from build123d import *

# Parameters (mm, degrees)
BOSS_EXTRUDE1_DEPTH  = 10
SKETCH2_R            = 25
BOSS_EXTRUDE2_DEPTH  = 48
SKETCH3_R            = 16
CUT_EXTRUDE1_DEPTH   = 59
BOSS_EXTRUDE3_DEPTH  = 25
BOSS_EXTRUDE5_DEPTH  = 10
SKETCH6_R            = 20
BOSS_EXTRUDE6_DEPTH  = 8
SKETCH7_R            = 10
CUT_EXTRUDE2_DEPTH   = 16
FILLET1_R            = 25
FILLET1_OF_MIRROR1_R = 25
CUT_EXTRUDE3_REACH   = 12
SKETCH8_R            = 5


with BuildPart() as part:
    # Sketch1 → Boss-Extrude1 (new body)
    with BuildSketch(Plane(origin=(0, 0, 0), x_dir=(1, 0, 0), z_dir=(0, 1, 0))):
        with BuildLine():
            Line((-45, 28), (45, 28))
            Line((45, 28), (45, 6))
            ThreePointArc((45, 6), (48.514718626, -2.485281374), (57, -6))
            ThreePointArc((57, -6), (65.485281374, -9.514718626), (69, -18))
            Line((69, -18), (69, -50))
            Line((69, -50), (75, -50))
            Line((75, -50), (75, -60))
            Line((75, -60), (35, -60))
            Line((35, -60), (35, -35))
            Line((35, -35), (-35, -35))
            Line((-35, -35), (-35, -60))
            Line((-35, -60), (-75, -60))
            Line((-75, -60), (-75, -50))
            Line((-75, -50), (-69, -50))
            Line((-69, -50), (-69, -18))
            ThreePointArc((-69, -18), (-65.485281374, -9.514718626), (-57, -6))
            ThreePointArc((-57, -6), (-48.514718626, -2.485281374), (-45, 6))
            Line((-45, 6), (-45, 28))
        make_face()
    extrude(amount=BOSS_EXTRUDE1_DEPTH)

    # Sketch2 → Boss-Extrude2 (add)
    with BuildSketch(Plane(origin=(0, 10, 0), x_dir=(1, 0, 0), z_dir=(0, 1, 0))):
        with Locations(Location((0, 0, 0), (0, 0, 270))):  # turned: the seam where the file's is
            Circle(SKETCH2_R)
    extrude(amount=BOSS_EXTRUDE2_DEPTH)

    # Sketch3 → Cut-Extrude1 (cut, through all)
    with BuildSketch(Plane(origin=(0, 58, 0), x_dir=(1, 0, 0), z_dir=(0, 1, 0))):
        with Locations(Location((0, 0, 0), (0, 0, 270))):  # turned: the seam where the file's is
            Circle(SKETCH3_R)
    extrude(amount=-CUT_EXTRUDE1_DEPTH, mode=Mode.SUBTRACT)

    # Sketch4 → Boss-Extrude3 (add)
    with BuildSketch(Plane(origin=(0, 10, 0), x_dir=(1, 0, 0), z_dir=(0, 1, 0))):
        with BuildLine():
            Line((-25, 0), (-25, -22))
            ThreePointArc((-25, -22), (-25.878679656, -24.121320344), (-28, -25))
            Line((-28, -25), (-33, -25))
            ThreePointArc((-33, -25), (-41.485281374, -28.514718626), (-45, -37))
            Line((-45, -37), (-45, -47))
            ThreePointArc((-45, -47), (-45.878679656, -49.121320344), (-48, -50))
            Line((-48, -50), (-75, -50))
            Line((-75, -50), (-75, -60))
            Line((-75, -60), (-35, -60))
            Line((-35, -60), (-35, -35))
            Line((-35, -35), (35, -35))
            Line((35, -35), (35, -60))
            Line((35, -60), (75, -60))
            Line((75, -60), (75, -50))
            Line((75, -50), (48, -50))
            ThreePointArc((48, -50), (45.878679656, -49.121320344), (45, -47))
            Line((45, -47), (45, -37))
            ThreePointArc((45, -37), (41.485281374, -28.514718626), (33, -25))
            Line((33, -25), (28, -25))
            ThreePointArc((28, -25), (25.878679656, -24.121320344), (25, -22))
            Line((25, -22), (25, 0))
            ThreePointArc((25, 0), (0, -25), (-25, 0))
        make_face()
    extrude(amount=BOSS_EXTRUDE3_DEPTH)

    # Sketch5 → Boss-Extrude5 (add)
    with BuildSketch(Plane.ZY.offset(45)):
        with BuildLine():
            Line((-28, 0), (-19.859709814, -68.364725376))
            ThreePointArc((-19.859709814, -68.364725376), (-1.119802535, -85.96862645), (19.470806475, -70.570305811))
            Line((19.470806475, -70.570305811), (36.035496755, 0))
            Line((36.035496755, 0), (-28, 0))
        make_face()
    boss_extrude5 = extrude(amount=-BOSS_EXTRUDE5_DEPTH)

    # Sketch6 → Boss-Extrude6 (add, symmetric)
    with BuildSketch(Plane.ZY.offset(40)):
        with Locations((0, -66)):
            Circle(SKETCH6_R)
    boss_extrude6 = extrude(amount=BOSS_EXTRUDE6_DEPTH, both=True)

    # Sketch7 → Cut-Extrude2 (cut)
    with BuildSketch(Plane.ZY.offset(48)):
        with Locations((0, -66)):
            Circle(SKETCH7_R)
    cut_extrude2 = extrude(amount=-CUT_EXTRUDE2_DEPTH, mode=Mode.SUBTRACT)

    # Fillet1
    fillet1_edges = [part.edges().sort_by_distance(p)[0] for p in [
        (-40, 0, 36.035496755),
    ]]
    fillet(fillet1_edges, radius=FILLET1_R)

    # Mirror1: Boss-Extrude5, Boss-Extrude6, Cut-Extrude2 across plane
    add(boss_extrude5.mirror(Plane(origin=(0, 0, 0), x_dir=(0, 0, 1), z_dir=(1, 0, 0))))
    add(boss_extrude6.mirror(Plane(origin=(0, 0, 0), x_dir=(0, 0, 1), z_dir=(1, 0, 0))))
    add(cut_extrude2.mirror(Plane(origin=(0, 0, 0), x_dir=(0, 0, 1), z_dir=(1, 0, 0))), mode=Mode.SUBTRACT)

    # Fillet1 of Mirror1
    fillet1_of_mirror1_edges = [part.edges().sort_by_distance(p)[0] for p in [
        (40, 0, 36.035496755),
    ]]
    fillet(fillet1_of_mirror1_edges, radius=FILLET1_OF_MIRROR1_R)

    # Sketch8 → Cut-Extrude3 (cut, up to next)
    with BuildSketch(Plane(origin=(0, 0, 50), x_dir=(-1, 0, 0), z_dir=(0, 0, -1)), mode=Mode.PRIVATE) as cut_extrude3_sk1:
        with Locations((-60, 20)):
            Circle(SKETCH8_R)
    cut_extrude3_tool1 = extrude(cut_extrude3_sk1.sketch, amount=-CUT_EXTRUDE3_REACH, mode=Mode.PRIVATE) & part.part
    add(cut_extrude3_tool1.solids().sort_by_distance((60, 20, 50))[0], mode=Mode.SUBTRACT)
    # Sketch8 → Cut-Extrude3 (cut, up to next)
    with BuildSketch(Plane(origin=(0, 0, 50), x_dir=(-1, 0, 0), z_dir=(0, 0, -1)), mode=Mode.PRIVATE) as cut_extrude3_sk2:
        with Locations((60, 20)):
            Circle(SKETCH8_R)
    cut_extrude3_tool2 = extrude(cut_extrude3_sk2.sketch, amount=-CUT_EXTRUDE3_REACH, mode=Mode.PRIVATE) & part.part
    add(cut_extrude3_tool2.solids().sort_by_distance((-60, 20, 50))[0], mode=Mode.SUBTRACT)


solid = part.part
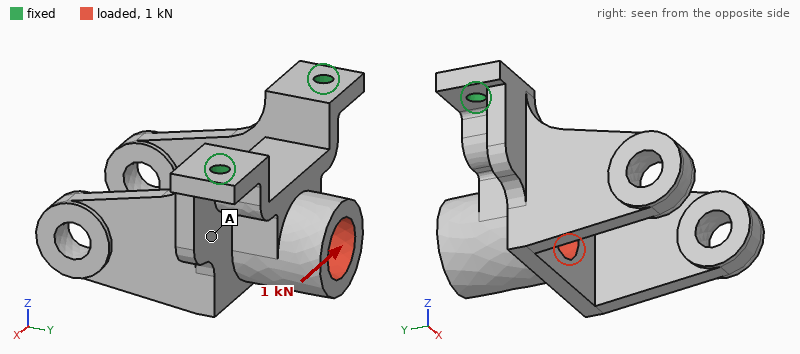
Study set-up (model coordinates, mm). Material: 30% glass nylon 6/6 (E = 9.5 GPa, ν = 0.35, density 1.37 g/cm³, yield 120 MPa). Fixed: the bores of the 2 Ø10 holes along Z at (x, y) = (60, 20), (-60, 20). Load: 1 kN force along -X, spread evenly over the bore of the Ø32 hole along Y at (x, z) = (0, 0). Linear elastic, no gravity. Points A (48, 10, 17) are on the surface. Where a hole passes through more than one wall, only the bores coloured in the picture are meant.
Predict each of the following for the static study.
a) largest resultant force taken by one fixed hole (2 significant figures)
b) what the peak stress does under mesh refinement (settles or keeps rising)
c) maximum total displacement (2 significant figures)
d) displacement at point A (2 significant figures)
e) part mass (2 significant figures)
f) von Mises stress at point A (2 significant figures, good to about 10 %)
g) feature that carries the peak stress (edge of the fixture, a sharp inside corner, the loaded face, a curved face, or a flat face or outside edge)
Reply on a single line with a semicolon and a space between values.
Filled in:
690 N; keeps rising; 80 µm; 36 µm; 380 g; 1.2 MPa; edge of the fixture
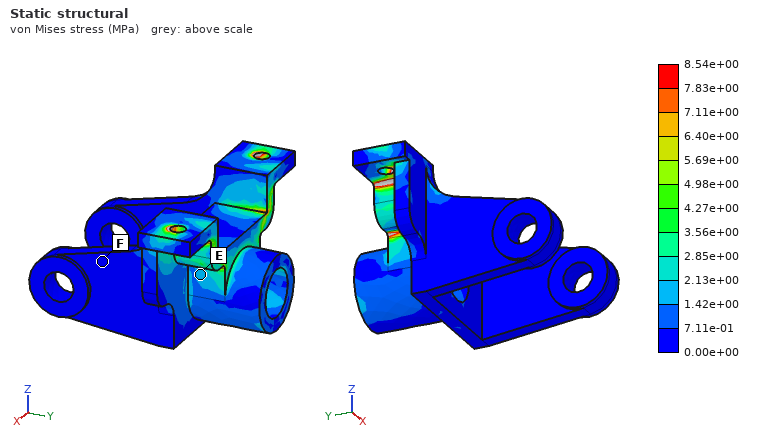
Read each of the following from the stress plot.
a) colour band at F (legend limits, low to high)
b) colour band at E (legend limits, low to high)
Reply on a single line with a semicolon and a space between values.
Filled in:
0.00e+00 to 7.11e-01 MPa; 1.42e+00 to 2.13e+00 MPa
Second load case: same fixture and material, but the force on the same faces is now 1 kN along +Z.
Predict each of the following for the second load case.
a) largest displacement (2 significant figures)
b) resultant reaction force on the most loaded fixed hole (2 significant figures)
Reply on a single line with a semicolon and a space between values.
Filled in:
0.25 mm; 610 N
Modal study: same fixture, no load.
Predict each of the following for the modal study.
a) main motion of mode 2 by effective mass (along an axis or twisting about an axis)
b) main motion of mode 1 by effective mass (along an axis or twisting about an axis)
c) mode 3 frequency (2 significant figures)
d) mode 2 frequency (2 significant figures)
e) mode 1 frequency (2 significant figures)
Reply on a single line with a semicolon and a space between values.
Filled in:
along X; along Y; 530 Hz; 500 Hz; 350 Hz
